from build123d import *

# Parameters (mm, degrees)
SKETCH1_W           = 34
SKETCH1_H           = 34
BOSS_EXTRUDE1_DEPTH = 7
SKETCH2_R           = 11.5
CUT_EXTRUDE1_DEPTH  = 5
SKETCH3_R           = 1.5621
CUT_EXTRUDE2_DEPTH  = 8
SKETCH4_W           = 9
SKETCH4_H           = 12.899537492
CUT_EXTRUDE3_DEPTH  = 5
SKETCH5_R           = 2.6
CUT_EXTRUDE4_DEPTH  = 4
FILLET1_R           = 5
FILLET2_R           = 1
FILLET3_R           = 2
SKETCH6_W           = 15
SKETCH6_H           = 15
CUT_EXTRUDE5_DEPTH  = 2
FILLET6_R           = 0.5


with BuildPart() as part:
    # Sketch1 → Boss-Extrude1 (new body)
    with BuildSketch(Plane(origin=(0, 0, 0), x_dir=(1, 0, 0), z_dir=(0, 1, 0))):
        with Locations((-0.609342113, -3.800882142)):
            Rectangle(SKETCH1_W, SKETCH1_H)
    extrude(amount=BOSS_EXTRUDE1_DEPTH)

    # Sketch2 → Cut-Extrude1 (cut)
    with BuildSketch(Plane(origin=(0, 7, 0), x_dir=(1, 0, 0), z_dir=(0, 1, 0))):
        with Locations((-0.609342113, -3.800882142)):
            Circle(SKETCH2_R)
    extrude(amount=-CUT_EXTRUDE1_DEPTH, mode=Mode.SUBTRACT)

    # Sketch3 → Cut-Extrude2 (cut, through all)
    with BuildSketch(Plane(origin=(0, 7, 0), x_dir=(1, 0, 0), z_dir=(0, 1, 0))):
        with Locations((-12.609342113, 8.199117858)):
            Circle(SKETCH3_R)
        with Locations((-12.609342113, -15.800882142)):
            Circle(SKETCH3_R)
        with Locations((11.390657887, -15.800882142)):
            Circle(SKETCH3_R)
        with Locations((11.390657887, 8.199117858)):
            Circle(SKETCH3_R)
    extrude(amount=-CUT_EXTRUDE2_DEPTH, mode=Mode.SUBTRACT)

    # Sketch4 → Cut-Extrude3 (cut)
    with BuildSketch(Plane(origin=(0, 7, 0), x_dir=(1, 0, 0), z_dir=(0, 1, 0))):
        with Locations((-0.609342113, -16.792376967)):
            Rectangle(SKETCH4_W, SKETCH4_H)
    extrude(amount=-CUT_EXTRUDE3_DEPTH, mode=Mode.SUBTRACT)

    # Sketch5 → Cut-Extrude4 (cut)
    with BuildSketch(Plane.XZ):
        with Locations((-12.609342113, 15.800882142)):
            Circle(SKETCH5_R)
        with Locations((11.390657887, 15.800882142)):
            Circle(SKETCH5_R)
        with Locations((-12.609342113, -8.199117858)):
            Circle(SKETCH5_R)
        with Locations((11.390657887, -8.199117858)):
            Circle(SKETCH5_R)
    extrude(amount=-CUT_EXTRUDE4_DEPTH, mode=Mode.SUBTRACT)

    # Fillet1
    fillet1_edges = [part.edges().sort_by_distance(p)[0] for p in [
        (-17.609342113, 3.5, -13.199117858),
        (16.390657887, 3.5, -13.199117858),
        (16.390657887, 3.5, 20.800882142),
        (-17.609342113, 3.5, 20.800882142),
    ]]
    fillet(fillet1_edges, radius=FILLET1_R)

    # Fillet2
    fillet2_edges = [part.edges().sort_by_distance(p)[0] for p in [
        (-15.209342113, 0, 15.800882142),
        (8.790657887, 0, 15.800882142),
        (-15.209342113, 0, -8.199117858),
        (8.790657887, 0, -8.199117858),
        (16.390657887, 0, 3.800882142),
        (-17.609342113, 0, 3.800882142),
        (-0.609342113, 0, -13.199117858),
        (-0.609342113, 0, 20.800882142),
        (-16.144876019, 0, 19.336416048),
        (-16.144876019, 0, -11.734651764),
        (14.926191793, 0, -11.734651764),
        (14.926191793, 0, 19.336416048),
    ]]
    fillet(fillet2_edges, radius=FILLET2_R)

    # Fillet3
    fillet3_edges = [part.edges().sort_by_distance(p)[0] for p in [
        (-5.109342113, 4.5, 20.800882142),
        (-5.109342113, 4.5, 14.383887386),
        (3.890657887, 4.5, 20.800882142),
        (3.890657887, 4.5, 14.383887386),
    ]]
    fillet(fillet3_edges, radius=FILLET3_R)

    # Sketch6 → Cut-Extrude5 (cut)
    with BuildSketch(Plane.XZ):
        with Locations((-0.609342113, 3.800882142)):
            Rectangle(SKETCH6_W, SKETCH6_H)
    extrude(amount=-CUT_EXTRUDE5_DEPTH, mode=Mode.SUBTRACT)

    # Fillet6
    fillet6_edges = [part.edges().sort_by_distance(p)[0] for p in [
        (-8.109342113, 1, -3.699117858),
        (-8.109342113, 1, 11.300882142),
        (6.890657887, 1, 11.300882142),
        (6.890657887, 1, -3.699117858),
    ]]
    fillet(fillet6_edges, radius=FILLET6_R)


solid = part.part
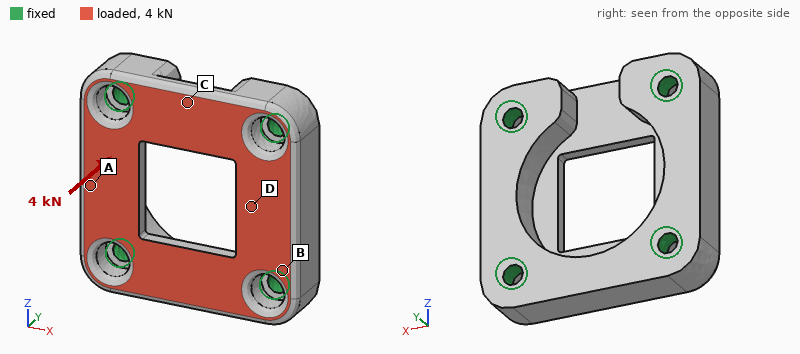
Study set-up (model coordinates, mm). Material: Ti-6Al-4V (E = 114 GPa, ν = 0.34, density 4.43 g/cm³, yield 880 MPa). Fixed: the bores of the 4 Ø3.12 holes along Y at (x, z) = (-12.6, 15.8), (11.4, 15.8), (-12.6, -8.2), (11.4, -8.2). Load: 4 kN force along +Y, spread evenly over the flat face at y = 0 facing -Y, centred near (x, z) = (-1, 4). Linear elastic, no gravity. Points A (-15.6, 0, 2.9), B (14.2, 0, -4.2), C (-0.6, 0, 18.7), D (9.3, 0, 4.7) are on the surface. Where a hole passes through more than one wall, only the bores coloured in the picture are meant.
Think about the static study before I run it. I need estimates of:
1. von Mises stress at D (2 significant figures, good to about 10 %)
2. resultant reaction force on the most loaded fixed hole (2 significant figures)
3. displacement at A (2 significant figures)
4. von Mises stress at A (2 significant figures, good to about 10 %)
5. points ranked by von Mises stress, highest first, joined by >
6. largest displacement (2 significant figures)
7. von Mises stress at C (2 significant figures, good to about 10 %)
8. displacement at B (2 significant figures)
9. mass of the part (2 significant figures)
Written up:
47 MPa
1.2 kN
4.5 µm
32 MPa
C > D > A > B
16 µm
65 MPa
2.9 µm
21 g
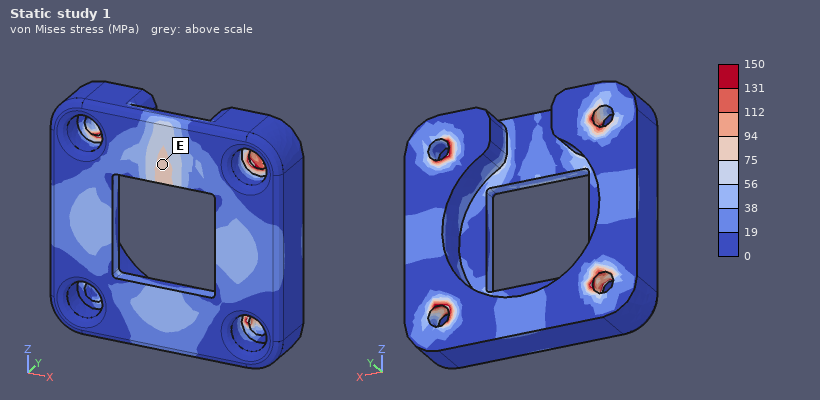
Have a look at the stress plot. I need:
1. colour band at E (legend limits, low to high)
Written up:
75 to 94 MPa
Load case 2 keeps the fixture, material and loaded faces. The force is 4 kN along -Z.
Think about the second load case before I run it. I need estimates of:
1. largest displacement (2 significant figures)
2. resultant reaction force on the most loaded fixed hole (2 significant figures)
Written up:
13 µm
1.1 kN
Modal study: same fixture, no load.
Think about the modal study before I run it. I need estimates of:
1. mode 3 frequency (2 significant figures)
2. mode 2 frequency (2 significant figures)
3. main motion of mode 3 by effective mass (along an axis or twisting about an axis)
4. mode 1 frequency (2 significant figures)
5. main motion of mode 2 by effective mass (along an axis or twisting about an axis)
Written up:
37 kHz
34 kHz
along Y
31 kHz
along X
